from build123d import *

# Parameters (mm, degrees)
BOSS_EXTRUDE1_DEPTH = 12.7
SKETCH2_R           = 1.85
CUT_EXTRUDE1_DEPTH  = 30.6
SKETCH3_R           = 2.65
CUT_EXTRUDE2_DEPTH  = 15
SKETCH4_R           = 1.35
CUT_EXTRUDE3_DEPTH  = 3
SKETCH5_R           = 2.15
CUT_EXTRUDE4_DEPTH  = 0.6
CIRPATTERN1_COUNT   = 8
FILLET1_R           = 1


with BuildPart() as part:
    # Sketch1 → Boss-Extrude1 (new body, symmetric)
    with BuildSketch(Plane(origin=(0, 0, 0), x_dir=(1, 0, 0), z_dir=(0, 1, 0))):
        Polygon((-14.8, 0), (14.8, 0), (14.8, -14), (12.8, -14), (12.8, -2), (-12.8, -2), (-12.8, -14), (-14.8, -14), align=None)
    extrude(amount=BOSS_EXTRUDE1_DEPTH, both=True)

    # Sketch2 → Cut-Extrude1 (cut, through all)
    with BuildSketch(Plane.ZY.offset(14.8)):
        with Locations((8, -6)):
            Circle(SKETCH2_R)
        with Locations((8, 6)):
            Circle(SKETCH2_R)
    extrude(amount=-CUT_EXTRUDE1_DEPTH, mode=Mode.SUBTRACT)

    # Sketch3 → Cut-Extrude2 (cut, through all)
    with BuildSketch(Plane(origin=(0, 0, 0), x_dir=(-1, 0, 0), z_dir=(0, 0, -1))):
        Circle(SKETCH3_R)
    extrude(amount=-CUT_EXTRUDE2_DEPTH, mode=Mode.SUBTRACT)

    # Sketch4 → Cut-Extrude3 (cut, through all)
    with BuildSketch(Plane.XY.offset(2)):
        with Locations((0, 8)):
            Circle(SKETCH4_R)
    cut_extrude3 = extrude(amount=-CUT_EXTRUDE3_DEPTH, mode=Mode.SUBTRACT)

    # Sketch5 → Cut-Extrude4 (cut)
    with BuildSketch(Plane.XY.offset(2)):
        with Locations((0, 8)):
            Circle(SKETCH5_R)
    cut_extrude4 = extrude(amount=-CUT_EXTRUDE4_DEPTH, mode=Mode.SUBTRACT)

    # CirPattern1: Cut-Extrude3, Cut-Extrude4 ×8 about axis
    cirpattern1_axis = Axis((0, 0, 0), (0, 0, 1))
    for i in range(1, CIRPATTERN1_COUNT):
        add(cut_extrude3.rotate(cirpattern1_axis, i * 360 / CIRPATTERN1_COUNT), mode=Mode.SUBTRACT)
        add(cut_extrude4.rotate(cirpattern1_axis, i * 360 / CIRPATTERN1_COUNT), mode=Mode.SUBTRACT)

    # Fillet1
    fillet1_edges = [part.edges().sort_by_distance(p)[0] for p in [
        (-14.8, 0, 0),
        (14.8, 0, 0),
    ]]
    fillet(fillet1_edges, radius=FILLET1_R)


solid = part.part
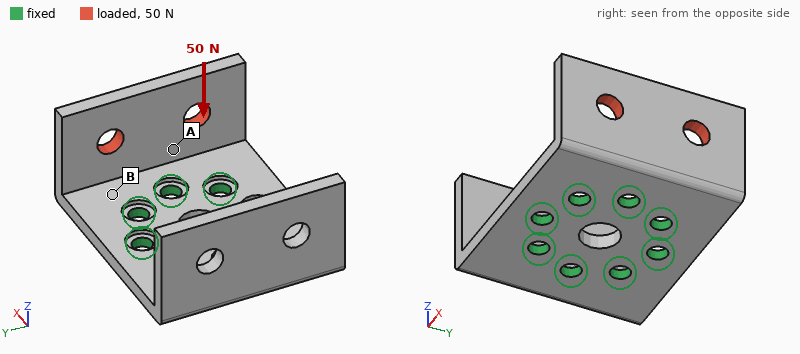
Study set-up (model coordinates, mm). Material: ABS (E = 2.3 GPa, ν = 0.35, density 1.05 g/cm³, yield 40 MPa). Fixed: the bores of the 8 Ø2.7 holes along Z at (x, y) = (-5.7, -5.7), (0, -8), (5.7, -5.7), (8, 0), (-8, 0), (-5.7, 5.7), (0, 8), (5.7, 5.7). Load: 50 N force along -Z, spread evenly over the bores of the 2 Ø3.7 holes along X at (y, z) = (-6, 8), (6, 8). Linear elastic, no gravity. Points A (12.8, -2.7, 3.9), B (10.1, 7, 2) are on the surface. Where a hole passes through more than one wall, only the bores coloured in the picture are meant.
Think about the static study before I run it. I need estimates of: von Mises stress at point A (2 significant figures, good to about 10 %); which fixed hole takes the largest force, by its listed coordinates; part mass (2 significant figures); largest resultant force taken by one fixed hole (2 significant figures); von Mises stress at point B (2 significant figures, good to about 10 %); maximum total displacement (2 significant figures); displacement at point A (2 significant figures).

2.9 MPa
(8, 0)
2.6 g
48 N
7.6 MPa
0.47 mm
0.16 mm
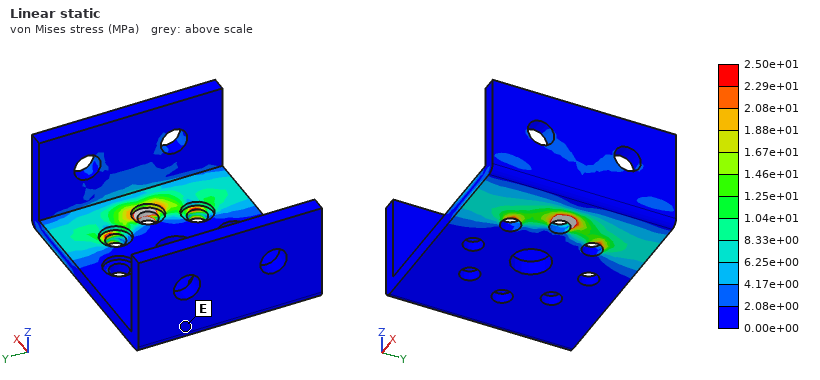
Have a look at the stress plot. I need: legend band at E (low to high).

0.00e+00 to 2.08e+00 MPa
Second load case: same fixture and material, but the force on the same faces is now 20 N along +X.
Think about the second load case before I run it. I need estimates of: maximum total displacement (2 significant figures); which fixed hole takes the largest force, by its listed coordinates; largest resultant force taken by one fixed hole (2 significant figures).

0.45 mm
(8, 0)
13 N
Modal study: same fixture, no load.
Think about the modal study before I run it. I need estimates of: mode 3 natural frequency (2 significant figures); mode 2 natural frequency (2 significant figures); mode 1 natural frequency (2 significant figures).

2200 Hz
1600 Hz
1600 Hz
